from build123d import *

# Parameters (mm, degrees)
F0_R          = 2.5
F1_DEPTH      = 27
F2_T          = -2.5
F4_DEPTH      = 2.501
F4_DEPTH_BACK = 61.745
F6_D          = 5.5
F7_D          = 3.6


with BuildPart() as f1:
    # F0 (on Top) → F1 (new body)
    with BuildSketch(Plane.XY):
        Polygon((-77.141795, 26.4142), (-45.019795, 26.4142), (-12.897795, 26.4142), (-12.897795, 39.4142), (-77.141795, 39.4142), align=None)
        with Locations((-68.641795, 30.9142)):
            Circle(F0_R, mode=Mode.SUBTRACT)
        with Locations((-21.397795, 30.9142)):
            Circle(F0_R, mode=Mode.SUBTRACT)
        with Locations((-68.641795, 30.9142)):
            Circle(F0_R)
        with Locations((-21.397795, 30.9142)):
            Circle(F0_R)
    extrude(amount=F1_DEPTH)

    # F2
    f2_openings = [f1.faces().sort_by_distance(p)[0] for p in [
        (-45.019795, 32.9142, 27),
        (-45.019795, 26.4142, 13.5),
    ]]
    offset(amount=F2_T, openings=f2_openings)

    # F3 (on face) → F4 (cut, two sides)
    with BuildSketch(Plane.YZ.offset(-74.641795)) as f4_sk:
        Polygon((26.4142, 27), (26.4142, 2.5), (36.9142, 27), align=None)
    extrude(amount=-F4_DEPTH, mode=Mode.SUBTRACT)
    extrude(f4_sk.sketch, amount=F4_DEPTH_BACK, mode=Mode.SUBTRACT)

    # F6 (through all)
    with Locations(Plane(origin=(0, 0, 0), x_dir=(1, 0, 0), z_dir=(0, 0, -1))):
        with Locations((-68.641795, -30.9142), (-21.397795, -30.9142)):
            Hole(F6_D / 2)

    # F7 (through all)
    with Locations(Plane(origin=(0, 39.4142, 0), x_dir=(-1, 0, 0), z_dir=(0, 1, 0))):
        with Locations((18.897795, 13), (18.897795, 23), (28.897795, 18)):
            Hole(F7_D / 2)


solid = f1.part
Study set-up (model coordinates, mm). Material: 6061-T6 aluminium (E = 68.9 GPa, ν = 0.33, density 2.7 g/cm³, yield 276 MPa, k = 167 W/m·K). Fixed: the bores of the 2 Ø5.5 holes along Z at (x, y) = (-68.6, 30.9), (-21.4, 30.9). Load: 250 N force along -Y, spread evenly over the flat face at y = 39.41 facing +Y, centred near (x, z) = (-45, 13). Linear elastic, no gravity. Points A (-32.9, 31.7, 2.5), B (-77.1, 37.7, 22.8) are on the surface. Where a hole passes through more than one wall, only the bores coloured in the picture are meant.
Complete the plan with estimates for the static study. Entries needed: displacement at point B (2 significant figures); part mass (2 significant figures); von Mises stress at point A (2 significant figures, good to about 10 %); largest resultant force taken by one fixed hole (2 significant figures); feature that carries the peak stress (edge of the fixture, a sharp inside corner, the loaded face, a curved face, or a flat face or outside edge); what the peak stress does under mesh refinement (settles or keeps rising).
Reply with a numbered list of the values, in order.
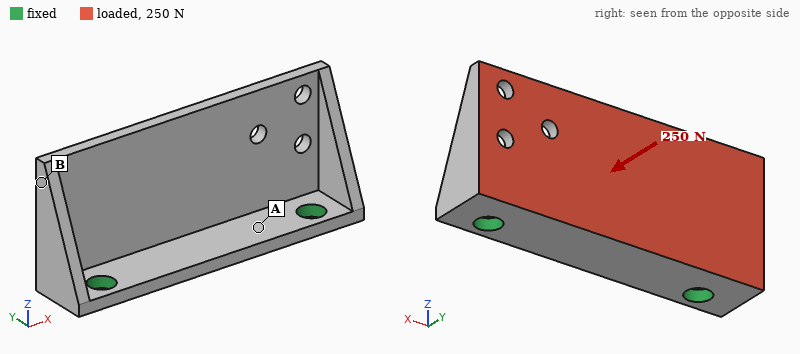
1. 0.042 mm
2. 17 g
3. 20 MPa
4. 130 N
5. edge of the fixture
6. keeps rising
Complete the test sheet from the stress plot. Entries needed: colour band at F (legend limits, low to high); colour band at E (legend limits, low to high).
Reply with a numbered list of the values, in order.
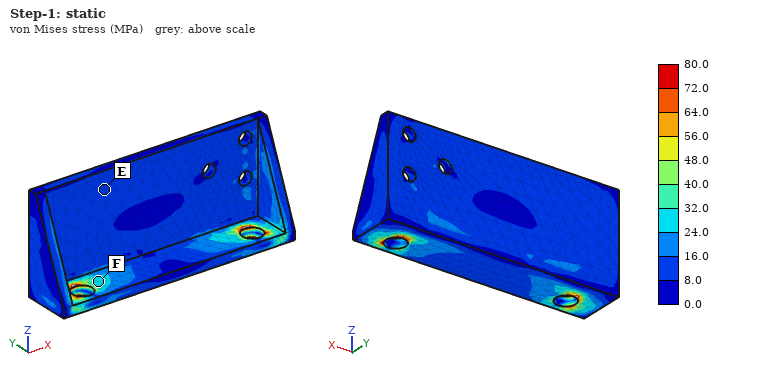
1. 24.0 to 32.0 MPa
2. 8.0 to 16.0 MPa
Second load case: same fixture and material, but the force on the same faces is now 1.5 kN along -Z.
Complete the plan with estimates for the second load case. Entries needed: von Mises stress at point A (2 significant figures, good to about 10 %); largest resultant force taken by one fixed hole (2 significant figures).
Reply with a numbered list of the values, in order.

1. 32 MPa
2. 770 N
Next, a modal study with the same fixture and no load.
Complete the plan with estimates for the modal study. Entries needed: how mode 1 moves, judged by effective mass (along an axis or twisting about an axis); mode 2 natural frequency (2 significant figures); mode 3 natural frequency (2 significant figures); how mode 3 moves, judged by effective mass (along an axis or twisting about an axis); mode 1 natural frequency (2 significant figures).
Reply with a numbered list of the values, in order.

1. along Y
2. 4900 Hz
3. 7600 Hz
4. along Z
5. 2800 Hz
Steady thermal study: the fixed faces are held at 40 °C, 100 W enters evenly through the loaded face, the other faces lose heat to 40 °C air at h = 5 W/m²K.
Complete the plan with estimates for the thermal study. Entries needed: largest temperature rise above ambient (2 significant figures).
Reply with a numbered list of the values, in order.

1. 83 K
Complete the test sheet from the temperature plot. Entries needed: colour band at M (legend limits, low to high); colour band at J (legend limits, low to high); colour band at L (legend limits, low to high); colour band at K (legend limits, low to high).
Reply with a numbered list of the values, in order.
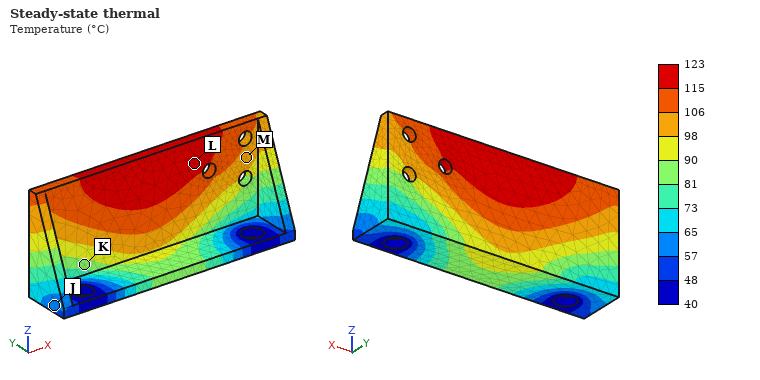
1. 98 to 106 °C
2. 57 to 65 °C
3. 115 to 123 °C
4. 81 to 90 °C
